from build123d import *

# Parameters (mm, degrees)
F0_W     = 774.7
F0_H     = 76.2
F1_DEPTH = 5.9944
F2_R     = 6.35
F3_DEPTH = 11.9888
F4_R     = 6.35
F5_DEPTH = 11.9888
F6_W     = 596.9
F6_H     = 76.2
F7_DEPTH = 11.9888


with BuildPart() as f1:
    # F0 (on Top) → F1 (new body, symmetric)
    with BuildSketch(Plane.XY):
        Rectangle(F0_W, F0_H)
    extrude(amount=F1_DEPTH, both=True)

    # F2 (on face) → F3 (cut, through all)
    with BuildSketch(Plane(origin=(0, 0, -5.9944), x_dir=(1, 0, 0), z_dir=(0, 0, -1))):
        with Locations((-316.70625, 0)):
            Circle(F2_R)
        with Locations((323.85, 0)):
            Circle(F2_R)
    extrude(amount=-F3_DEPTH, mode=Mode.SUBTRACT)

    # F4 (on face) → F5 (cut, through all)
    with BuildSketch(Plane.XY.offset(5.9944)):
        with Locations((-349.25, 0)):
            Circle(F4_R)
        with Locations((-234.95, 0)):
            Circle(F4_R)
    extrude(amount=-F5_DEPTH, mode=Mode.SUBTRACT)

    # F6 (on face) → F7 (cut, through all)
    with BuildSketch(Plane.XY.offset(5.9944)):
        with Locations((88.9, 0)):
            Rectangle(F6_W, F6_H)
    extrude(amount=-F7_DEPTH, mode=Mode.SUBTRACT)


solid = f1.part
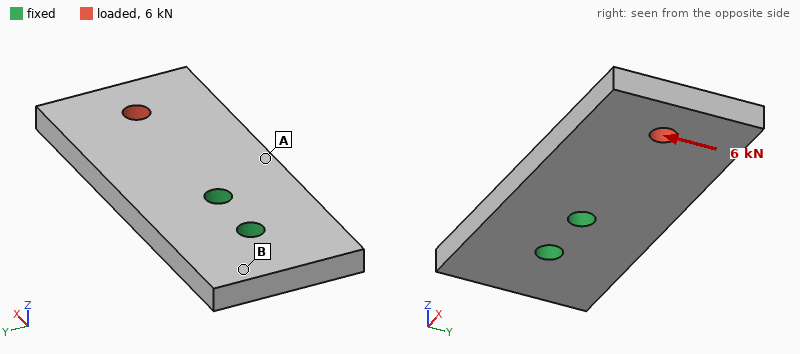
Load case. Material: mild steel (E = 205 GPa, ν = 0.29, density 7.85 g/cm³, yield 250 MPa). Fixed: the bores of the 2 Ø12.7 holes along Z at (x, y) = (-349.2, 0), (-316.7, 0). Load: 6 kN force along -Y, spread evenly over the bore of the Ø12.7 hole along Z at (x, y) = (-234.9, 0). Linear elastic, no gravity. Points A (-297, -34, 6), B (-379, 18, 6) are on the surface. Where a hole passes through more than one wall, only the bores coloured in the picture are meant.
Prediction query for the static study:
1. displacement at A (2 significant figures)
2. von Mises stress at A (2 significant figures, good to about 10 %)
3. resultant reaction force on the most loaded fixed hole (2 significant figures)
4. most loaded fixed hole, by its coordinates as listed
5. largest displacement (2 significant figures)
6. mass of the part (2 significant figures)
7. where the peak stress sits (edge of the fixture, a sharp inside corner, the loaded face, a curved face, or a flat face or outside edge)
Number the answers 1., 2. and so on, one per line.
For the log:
1. 14 µm
2. 30 MPa
3. 16 kN
4. (-316.7, 0)
5. 55 µm
6. 1.2 kg
7. edge of the fixture
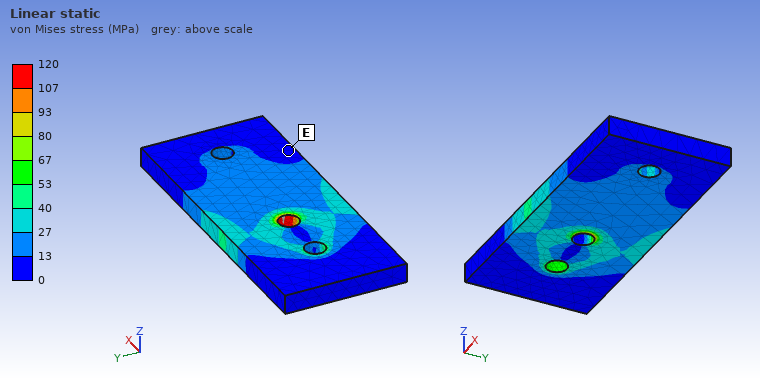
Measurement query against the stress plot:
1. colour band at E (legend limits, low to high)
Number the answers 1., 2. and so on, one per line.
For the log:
1. 0 to 13 MPa
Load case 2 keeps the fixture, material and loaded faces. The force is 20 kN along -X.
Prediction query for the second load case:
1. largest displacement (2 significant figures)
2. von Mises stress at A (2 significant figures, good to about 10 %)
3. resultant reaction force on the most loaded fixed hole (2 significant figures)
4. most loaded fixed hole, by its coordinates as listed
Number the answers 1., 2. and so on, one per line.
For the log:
1. 15 µm
2. 15 MPa
3. 15 kN
4. (-316.7, 0)
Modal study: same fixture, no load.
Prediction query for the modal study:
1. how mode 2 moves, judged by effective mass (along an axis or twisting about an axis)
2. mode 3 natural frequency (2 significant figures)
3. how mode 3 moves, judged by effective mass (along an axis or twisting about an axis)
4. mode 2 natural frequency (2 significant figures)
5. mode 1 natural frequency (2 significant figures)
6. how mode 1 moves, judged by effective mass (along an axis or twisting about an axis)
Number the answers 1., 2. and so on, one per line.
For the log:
1. twisting about X
2. 2900 Hz
3. along Y
4. 2200 Hz
5. 870 Hz
6. along Z
